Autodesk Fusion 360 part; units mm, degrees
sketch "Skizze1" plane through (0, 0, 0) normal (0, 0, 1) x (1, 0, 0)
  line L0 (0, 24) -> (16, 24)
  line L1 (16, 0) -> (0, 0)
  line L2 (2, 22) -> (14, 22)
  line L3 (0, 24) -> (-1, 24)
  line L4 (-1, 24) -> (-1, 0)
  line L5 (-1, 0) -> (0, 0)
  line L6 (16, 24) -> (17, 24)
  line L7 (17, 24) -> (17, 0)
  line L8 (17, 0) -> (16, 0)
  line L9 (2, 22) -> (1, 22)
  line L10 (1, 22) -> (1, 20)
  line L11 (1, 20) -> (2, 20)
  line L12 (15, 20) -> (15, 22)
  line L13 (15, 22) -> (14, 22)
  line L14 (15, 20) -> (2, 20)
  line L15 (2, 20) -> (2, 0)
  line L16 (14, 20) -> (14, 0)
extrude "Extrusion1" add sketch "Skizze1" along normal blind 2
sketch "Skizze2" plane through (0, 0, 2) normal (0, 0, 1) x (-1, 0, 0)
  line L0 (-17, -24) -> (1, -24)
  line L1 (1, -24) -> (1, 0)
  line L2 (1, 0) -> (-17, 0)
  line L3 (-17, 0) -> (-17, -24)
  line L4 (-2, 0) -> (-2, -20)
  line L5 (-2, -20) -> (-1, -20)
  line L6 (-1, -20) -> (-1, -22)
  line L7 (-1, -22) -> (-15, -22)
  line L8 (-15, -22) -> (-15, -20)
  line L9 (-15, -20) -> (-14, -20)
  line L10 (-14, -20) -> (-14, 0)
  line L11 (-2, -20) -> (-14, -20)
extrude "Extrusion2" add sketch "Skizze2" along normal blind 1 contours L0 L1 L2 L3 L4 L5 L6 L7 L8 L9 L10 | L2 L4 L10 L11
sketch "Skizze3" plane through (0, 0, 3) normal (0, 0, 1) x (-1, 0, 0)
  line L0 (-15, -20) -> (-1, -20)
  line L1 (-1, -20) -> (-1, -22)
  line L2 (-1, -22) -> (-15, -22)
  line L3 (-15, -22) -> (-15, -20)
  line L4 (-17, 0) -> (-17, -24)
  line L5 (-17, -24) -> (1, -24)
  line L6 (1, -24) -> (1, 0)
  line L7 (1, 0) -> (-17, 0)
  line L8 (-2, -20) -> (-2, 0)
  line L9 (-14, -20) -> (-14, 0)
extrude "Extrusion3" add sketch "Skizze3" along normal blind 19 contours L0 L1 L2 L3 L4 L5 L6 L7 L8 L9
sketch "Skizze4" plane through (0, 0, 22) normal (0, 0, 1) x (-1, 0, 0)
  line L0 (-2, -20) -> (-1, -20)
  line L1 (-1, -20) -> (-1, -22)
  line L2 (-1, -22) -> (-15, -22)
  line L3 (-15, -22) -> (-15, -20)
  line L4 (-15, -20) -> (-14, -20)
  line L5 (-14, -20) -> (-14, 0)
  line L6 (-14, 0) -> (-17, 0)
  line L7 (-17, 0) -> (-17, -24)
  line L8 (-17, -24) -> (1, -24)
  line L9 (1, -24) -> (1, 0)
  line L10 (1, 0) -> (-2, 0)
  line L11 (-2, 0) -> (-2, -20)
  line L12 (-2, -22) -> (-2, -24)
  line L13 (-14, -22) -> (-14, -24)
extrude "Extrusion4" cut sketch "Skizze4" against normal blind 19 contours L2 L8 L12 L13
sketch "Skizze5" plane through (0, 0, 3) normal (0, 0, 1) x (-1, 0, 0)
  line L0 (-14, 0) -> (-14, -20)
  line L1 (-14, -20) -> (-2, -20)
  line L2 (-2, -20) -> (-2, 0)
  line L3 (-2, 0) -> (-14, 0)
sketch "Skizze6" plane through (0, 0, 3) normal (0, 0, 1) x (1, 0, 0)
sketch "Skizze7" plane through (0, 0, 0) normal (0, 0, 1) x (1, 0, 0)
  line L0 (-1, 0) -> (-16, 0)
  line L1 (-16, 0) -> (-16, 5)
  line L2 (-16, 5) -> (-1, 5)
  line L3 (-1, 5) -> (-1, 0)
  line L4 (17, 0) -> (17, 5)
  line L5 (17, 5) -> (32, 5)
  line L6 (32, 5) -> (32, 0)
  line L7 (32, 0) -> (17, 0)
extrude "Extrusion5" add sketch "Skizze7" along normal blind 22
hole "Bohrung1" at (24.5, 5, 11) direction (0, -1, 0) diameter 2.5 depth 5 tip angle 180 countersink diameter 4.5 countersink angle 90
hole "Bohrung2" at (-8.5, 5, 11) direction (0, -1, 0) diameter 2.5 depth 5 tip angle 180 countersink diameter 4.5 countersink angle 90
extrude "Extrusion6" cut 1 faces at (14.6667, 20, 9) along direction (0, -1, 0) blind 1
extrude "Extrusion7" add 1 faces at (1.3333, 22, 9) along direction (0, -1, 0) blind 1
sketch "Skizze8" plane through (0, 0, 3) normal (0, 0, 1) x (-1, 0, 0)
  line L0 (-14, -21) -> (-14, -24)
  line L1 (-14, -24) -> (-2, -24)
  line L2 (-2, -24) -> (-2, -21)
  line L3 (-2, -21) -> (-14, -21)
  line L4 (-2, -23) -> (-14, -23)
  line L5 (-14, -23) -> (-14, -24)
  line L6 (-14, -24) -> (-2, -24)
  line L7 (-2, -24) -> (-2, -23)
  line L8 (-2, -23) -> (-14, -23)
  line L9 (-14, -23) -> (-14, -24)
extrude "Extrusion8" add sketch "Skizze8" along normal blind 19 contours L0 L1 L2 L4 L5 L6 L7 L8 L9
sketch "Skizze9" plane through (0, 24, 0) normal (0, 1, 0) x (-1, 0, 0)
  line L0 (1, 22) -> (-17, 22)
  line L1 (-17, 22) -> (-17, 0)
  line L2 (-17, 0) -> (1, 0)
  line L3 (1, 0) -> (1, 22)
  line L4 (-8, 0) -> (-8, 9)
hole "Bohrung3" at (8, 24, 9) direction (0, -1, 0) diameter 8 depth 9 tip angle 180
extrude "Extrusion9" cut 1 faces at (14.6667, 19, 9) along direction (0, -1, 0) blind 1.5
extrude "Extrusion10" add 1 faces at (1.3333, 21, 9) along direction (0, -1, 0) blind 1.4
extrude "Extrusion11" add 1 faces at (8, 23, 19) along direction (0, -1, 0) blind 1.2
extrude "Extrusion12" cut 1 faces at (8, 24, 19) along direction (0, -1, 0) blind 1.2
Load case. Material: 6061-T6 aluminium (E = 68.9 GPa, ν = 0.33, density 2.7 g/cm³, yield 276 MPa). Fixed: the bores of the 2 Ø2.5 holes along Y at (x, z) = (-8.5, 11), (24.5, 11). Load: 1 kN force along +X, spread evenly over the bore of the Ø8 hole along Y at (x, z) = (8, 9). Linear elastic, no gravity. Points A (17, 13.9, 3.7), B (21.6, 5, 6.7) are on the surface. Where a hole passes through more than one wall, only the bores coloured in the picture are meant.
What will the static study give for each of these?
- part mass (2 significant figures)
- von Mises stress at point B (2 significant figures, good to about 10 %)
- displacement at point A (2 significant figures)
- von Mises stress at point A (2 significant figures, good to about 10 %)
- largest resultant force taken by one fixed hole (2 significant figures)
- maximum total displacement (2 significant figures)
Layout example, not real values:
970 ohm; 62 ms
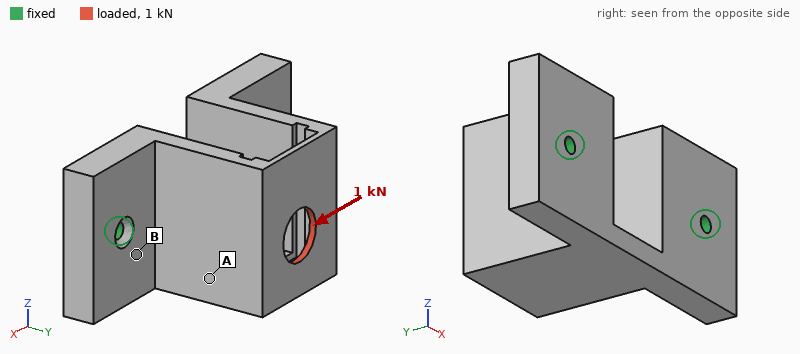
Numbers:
19 g; 25 MPa; 0.050 mm; 54 MPa; 780 N; 0.18 mm
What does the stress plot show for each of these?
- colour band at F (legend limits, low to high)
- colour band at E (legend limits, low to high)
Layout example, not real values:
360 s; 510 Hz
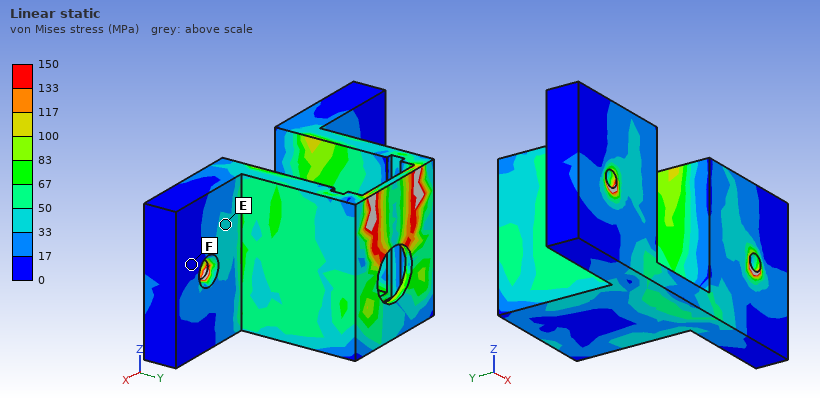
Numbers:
0 to 17 MPa; 33 to 50 MPa
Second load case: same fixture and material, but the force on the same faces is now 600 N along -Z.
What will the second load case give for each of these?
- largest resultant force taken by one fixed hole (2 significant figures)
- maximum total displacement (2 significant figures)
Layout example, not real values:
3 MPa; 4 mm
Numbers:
370 N; 0.10 mm
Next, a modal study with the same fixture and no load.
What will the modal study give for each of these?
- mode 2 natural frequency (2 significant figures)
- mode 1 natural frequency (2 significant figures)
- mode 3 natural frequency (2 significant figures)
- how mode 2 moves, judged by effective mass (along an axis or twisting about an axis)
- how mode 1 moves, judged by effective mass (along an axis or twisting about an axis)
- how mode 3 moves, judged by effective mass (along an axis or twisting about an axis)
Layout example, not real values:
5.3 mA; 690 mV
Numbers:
7100 Hz; 5900 Hz; 12 kHz; along X; along Z; along Y
